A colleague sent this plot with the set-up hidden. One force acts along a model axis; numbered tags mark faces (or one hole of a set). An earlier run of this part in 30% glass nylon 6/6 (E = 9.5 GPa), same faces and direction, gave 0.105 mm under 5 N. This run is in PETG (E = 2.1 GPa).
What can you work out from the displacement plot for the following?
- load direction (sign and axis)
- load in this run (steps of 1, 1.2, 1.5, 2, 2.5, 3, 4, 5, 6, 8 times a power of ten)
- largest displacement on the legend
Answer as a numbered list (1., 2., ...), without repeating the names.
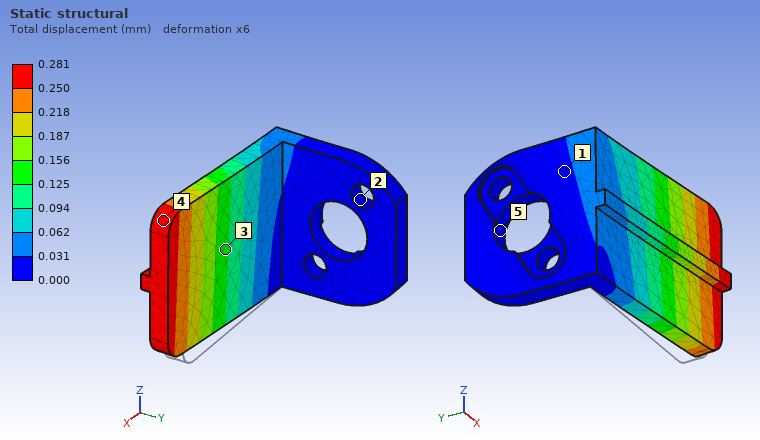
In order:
1. -Y
2. 3 N
3. 0.281 mm
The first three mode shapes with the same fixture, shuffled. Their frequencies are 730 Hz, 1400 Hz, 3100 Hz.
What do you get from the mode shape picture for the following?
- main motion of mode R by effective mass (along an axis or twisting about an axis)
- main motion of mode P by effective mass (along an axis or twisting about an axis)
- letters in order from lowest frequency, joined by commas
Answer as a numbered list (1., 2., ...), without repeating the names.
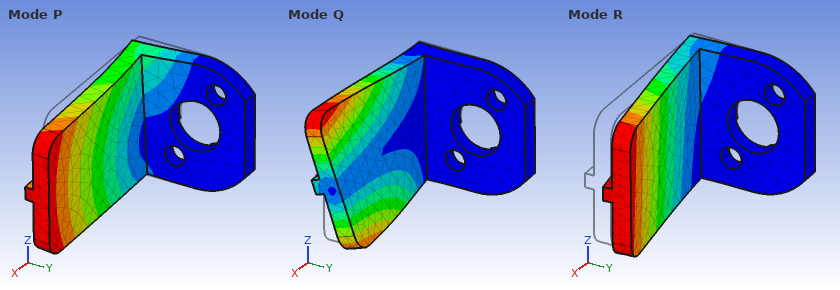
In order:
1. along Y
2. along Z
3. R, P, Q
